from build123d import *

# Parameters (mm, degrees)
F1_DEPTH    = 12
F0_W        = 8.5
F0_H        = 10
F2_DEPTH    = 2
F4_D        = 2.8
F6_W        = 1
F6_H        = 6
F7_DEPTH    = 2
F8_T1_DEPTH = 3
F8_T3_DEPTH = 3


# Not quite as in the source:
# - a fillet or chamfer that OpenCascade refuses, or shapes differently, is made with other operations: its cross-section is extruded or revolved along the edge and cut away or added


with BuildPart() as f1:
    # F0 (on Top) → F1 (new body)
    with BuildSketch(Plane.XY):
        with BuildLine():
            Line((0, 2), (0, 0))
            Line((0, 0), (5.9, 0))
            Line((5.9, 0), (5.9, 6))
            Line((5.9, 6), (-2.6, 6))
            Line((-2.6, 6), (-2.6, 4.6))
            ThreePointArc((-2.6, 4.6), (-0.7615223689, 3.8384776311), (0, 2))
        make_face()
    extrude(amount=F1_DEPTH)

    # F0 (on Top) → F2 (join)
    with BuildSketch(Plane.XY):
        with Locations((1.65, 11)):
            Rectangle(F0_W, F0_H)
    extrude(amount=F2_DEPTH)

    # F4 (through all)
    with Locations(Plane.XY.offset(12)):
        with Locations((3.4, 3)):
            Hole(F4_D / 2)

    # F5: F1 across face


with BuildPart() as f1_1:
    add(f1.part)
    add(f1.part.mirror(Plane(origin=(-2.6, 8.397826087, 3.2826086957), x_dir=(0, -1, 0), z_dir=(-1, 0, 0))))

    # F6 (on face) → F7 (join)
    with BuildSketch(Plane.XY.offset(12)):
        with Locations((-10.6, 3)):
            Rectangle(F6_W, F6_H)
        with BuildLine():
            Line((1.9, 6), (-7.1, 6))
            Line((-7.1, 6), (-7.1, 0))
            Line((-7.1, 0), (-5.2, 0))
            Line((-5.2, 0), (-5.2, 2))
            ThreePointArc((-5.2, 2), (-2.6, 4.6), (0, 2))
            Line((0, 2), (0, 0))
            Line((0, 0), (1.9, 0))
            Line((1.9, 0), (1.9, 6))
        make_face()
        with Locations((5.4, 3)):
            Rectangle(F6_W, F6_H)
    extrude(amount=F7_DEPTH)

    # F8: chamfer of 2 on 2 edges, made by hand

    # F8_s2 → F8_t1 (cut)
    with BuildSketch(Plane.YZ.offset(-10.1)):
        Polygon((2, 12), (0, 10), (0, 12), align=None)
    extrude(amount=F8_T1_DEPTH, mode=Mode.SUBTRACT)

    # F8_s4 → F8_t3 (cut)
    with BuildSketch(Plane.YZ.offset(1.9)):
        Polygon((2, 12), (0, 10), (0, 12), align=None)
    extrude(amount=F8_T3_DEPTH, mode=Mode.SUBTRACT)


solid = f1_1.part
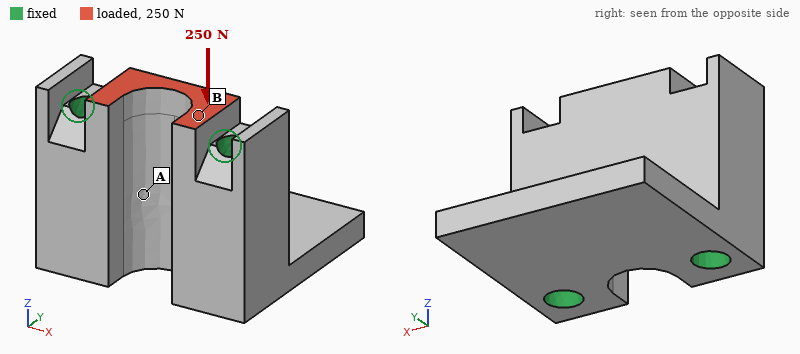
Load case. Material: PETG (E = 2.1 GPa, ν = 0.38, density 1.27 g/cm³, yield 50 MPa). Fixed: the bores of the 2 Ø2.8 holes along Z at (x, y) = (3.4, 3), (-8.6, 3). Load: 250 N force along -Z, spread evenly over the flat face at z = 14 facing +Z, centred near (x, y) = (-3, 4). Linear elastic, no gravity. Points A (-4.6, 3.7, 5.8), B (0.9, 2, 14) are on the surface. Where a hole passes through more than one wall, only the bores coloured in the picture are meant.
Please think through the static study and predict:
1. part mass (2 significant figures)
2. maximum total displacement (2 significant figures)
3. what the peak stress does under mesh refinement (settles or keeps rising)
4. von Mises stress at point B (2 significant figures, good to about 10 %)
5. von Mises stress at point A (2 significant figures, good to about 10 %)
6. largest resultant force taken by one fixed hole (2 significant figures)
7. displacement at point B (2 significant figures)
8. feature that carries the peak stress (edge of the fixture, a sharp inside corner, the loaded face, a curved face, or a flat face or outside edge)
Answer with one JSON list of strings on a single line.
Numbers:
["1.6 g", "34 µm", "keeps rising", "8.4 MPa", "2.3 MPa", "130 N", "23 µm", "edge of the fixture"]
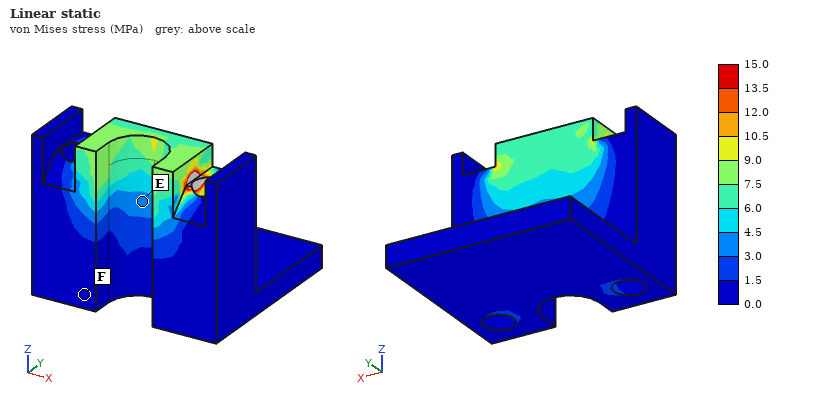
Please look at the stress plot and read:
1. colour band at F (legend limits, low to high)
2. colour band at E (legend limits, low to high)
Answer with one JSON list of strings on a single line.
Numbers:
["0.0 to 1.5 MPa", "3.0 to 4.5 MPa"]
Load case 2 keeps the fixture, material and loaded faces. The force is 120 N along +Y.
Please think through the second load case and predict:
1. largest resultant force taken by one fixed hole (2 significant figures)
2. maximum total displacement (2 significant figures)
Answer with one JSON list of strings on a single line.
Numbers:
["61 N", "74 µm"]
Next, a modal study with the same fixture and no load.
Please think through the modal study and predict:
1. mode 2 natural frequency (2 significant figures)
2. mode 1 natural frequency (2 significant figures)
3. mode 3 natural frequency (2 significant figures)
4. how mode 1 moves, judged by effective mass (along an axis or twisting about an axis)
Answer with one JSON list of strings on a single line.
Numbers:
["5800 Hz", "3400 Hz", "13 kHz", "along Z"]
